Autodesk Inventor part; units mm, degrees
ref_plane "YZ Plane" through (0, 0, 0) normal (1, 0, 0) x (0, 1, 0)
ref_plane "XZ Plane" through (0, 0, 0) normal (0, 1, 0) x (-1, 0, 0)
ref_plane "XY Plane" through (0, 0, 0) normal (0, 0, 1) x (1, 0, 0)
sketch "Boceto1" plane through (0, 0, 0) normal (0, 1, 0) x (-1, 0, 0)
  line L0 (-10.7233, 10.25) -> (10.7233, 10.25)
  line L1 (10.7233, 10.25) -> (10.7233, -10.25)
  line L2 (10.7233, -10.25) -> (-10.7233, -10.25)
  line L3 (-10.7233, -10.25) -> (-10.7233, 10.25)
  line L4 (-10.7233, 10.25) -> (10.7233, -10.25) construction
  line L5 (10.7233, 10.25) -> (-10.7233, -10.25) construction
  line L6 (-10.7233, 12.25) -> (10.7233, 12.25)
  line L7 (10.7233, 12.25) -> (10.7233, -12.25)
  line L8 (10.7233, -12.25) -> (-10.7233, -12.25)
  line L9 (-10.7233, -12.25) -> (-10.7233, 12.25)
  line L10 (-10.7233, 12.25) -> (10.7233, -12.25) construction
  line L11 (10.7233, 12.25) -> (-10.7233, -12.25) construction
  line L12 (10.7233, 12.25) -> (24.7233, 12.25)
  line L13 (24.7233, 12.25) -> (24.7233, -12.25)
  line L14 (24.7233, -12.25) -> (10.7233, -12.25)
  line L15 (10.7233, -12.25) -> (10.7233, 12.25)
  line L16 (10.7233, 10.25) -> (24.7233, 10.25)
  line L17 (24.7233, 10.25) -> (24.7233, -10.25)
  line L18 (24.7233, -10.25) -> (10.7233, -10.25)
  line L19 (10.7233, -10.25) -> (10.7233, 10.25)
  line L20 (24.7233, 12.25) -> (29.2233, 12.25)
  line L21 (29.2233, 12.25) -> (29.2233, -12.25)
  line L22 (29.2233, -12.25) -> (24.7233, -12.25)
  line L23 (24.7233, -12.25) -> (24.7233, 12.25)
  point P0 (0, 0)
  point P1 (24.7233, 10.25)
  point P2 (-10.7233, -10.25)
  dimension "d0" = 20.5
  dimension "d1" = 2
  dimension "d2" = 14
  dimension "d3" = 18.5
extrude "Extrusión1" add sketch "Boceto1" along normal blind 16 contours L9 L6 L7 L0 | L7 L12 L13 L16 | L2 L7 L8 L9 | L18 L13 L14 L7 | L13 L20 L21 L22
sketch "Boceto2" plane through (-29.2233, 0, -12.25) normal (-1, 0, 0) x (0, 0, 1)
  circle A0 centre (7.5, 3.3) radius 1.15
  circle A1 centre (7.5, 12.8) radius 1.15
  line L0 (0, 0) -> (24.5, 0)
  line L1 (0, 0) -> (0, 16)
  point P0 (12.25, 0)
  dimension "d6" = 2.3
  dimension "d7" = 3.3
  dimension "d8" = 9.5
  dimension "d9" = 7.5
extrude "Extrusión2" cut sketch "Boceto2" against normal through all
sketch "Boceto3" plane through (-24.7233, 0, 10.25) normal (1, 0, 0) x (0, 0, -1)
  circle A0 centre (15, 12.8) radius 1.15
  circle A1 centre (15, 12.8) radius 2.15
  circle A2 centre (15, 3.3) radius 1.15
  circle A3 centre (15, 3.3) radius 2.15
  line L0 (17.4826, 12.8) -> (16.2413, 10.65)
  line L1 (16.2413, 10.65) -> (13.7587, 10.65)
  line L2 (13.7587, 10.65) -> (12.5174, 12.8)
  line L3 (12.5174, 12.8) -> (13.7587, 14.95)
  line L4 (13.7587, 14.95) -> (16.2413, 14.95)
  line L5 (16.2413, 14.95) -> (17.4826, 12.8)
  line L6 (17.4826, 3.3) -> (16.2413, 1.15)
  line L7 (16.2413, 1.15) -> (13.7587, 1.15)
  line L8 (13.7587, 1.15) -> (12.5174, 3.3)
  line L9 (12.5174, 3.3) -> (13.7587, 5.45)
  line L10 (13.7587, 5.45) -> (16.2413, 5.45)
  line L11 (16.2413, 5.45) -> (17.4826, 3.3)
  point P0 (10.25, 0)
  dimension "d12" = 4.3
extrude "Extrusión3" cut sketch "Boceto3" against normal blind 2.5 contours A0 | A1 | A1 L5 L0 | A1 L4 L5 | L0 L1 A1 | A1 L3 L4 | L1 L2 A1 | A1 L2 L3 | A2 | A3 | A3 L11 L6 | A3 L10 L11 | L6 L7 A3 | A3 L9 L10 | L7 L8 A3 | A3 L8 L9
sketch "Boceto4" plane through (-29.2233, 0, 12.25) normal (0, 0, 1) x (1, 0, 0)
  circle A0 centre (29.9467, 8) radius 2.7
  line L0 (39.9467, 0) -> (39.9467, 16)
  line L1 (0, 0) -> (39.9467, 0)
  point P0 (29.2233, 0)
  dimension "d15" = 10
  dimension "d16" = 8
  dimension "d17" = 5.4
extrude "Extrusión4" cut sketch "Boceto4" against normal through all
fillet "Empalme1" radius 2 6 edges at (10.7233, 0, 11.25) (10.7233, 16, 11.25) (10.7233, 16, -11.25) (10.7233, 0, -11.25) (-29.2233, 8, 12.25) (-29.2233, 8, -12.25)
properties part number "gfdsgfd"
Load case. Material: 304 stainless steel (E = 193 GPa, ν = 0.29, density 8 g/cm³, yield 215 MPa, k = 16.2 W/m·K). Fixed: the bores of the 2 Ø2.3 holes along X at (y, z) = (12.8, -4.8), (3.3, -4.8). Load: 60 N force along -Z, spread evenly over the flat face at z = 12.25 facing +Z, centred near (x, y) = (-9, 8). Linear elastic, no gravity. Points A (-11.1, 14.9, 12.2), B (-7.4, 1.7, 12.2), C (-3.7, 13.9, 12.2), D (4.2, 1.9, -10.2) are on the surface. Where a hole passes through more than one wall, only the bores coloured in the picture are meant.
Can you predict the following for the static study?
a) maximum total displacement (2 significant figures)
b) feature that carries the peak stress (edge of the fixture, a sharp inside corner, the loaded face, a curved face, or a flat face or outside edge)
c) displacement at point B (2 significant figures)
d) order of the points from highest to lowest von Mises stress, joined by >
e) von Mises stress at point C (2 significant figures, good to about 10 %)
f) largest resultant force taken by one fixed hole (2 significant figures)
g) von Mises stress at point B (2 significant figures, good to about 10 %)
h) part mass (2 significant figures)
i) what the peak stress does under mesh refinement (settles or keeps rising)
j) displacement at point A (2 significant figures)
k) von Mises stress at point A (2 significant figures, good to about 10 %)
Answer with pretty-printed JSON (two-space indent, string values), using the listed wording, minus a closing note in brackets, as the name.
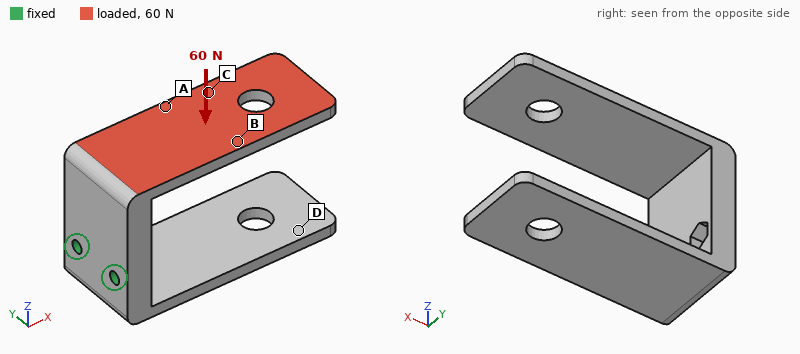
{
  "maximum total displacement": "0.20 mm",
  "feature that carries the peak stress": "edge of the fixture",
  "displacement at point B": "0.081 mm",
  "order of the points from highest to lowest von Mises stress, joined by >": "A > B > C > D",
  "von Mises stress at point C": "17 MPa",
  "largest resultant force taken by one fixed hole": "35 N",
  "von Mises stress at point B": "24 MPa",
  "part mass": "30 g",
  "what the peak stress does under mesh refinement": "keeps rising",
  "displacement at point A": "0.059 mm",
  "von Mises stress at point A": "34 MPa"
}
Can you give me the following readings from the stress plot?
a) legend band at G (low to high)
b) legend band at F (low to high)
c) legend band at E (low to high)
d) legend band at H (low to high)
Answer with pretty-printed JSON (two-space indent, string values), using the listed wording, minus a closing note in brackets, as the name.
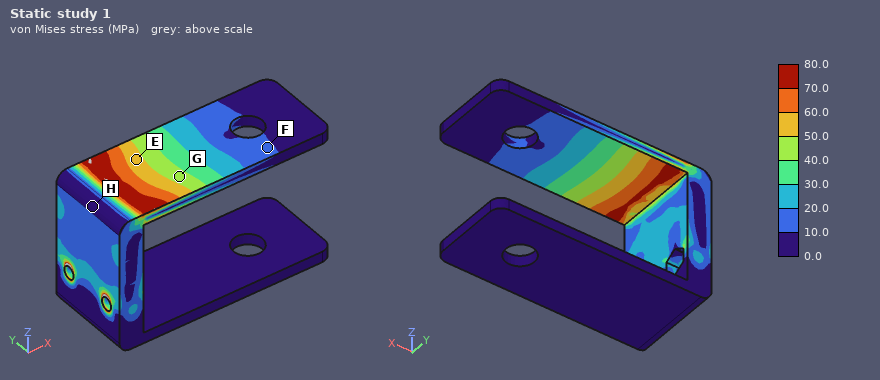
{
  "legend band at G": "40.0 to 50.0 MPa",
  "legend band at F": "10.0 to 20.0 MPa",
  "legend band at E": "50.0 to 60.0 MPa",
  "legend band at H": "0.0 to 10.0 MPa"
}
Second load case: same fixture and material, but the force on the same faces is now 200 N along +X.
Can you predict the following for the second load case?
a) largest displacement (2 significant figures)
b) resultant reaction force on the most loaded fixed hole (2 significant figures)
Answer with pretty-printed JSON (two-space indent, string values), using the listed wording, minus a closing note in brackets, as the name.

{
  "largest displacement": "0.14 mm",
  "resultant reaction force on the most loaded fixed hole": "110 N"
}
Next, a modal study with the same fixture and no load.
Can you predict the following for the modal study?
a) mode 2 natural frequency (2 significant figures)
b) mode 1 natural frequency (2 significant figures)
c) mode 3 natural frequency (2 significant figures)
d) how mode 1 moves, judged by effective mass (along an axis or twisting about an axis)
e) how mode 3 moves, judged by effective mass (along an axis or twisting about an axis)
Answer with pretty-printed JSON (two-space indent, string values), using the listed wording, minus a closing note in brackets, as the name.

{
  "mode 2 natural frequency": "1200 Hz",
  "mode 1 natural frequency": "1100 Hz",
  "mode 3 natural frequency": "3100 Hz",
  "how mode 1 moves, judged by effective mass": "along Z",
  "how mode 3 moves, judged by effective mass": "along Y"
}
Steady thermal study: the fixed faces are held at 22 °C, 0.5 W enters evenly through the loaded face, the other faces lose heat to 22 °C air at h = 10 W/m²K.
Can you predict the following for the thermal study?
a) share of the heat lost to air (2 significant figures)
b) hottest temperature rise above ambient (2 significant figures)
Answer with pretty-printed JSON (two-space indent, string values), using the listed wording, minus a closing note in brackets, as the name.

{
  "share of the heat lost to air": "28 %",
  "hottest temperature rise above ambient": "18 K"
}
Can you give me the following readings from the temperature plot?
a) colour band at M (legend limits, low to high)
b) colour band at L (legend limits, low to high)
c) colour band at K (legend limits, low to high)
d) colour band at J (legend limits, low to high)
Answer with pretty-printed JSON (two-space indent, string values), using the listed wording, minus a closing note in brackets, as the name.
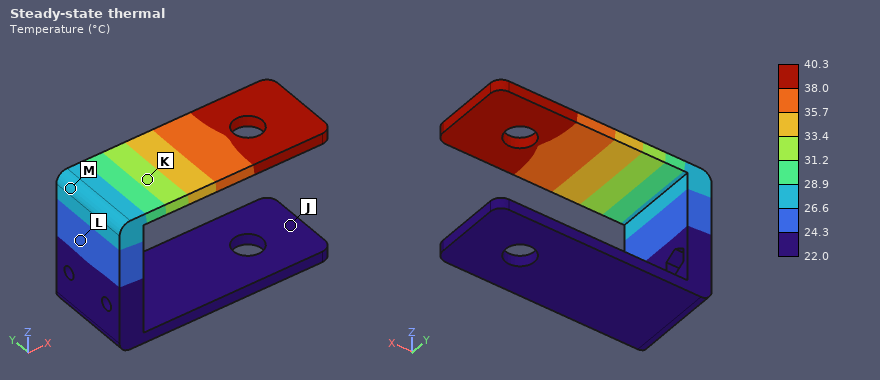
{
  "colour band at M": "26.6 to 28.9 °C",
  "colour band at L": "24.3 to 26.6 °C",
  "colour band at K": "31.2 to 33.4 °C",
  "colour band at J": "22.0 to 24.3 °C"
}
